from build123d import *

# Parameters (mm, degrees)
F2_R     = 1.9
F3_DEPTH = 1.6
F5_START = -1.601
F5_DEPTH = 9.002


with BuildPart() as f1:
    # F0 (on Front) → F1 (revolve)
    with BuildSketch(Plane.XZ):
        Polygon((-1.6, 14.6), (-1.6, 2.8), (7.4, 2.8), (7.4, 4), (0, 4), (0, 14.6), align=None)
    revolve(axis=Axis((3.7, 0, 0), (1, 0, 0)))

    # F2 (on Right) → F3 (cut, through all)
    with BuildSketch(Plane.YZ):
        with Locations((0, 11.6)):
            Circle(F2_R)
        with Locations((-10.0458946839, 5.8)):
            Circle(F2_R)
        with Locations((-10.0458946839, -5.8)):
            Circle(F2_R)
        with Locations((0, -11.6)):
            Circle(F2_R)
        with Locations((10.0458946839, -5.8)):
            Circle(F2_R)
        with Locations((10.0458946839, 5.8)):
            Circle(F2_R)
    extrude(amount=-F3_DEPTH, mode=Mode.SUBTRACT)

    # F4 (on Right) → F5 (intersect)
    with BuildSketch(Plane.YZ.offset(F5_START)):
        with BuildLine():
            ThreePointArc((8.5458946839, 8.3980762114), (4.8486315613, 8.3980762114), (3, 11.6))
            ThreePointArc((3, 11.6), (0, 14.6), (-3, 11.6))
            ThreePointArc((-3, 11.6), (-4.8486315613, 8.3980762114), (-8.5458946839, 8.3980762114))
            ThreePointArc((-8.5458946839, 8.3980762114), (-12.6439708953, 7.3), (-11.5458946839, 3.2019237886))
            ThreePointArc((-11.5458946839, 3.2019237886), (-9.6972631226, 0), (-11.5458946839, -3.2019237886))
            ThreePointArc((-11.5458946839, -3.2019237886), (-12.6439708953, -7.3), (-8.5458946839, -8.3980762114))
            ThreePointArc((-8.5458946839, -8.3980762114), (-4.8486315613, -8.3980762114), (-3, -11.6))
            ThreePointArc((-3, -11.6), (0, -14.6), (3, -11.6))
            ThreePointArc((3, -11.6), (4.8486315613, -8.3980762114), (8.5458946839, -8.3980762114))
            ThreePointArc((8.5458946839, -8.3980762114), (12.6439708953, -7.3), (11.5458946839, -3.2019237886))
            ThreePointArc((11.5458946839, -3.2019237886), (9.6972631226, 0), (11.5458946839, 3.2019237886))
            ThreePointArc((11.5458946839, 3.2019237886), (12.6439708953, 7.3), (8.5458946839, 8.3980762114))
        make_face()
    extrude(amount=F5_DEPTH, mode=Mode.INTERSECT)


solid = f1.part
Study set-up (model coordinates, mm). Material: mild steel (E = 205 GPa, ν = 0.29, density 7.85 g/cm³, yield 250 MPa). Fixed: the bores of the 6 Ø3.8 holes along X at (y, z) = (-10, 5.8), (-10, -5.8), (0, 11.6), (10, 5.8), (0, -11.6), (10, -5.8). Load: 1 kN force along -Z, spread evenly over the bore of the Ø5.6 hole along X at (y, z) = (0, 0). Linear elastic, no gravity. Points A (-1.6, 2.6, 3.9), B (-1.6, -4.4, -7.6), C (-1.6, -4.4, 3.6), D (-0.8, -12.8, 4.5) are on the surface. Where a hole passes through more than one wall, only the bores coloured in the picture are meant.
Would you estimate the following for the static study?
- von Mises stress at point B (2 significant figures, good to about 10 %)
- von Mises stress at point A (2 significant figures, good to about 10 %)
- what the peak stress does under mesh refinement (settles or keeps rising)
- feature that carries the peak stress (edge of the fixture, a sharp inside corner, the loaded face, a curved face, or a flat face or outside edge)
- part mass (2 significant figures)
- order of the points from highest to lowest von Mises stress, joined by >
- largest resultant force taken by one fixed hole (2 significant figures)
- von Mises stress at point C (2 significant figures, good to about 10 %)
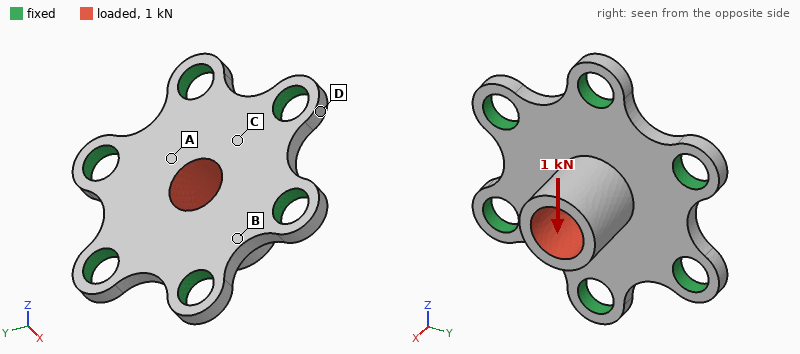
35 MPa
91 MPa
keeps rising
edge of the fixture
6.2 g
A > C > B > D
330 N
64 MPa
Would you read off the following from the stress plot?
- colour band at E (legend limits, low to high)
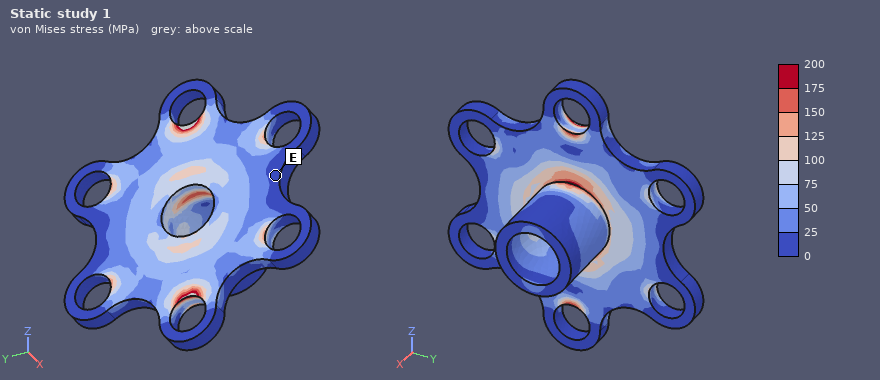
0 to 25 MPa
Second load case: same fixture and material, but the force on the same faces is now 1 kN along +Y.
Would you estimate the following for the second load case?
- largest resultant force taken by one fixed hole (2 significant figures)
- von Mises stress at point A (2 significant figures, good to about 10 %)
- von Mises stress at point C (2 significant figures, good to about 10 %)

290 N
77 MPa
68 MPa
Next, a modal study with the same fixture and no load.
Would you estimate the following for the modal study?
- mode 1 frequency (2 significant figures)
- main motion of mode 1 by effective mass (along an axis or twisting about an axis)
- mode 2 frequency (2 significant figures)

26 kHz
along X
28 kHz
